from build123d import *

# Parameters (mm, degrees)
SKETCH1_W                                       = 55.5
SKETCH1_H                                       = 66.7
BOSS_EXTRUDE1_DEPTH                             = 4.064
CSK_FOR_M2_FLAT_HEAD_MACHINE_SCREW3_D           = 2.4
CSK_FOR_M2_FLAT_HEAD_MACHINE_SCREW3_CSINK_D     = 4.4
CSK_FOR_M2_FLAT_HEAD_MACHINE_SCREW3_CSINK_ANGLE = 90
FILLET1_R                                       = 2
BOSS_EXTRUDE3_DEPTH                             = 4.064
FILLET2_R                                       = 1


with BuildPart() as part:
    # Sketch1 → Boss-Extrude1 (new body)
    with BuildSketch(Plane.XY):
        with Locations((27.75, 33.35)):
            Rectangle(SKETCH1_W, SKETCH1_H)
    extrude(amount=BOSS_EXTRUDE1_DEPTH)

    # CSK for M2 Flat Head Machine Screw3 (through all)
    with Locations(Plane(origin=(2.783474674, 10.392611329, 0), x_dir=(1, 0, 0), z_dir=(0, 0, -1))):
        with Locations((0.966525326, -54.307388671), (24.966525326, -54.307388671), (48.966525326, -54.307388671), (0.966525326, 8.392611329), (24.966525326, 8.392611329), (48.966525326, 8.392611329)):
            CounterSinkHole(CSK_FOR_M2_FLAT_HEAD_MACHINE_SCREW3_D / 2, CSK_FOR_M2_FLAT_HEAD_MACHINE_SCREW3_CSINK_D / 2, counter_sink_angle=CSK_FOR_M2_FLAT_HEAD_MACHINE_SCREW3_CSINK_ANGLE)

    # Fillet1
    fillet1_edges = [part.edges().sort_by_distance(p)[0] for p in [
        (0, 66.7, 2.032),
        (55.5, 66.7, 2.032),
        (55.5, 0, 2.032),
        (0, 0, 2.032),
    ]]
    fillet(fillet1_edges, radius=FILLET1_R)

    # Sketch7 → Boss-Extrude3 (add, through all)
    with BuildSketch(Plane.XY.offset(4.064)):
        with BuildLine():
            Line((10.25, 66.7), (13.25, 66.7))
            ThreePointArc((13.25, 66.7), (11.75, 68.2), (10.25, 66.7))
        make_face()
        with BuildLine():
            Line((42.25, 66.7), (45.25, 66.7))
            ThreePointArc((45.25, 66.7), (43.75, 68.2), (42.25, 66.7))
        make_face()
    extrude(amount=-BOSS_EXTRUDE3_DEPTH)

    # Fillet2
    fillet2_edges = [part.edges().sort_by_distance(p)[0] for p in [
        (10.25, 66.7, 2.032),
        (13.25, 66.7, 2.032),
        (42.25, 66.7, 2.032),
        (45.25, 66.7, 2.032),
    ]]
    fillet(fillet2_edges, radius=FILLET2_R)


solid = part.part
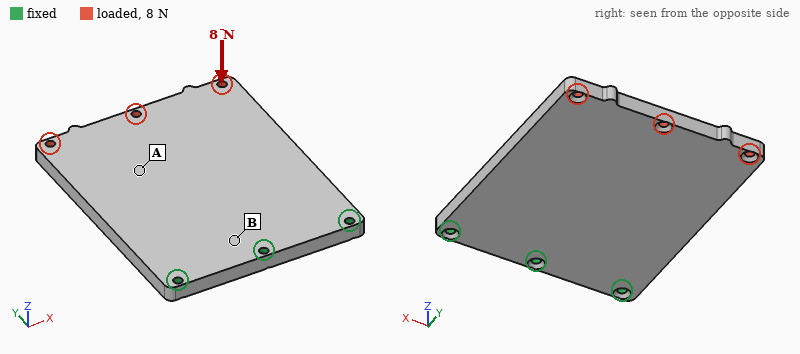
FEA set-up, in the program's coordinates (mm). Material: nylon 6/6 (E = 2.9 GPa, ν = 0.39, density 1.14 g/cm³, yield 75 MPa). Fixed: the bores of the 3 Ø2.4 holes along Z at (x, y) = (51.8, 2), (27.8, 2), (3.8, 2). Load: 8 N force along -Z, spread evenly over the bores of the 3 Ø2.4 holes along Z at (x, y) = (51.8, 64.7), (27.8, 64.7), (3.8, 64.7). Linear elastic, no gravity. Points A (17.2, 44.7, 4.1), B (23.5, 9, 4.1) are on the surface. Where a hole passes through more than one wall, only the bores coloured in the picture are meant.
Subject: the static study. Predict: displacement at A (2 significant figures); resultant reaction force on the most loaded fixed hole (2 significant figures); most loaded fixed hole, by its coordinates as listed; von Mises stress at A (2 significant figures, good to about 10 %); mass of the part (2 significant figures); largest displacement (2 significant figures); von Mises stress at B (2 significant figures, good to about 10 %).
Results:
0.54 mm
8.2 N
(27.8, 2)
1.0 MPa
17 g
1.0 mm
2.7 MPa
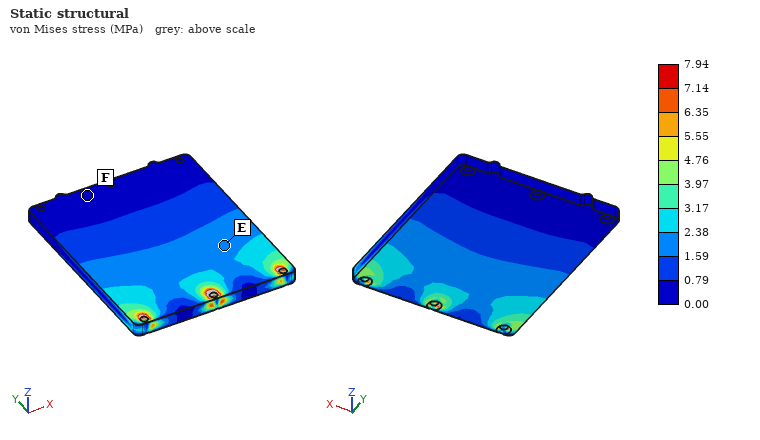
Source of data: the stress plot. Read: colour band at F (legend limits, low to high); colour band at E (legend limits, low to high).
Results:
0.00 to 0.79 MPa
1.59 to 2.38 MPa
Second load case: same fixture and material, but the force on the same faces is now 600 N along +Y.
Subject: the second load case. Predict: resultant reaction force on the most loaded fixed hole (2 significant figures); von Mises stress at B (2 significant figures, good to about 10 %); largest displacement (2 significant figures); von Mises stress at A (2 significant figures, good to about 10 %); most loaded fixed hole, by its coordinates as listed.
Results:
230 N
5.0 MPa
0.75 mm
4.0 MPa
(27.8, 2)
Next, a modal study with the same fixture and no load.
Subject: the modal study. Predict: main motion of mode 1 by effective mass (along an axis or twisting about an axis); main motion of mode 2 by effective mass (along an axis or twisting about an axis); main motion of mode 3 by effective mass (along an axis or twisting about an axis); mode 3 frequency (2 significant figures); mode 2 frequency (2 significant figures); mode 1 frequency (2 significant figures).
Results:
along Z
twisting about Y
along Z
1400 Hz
650 Hz
210 Hz
